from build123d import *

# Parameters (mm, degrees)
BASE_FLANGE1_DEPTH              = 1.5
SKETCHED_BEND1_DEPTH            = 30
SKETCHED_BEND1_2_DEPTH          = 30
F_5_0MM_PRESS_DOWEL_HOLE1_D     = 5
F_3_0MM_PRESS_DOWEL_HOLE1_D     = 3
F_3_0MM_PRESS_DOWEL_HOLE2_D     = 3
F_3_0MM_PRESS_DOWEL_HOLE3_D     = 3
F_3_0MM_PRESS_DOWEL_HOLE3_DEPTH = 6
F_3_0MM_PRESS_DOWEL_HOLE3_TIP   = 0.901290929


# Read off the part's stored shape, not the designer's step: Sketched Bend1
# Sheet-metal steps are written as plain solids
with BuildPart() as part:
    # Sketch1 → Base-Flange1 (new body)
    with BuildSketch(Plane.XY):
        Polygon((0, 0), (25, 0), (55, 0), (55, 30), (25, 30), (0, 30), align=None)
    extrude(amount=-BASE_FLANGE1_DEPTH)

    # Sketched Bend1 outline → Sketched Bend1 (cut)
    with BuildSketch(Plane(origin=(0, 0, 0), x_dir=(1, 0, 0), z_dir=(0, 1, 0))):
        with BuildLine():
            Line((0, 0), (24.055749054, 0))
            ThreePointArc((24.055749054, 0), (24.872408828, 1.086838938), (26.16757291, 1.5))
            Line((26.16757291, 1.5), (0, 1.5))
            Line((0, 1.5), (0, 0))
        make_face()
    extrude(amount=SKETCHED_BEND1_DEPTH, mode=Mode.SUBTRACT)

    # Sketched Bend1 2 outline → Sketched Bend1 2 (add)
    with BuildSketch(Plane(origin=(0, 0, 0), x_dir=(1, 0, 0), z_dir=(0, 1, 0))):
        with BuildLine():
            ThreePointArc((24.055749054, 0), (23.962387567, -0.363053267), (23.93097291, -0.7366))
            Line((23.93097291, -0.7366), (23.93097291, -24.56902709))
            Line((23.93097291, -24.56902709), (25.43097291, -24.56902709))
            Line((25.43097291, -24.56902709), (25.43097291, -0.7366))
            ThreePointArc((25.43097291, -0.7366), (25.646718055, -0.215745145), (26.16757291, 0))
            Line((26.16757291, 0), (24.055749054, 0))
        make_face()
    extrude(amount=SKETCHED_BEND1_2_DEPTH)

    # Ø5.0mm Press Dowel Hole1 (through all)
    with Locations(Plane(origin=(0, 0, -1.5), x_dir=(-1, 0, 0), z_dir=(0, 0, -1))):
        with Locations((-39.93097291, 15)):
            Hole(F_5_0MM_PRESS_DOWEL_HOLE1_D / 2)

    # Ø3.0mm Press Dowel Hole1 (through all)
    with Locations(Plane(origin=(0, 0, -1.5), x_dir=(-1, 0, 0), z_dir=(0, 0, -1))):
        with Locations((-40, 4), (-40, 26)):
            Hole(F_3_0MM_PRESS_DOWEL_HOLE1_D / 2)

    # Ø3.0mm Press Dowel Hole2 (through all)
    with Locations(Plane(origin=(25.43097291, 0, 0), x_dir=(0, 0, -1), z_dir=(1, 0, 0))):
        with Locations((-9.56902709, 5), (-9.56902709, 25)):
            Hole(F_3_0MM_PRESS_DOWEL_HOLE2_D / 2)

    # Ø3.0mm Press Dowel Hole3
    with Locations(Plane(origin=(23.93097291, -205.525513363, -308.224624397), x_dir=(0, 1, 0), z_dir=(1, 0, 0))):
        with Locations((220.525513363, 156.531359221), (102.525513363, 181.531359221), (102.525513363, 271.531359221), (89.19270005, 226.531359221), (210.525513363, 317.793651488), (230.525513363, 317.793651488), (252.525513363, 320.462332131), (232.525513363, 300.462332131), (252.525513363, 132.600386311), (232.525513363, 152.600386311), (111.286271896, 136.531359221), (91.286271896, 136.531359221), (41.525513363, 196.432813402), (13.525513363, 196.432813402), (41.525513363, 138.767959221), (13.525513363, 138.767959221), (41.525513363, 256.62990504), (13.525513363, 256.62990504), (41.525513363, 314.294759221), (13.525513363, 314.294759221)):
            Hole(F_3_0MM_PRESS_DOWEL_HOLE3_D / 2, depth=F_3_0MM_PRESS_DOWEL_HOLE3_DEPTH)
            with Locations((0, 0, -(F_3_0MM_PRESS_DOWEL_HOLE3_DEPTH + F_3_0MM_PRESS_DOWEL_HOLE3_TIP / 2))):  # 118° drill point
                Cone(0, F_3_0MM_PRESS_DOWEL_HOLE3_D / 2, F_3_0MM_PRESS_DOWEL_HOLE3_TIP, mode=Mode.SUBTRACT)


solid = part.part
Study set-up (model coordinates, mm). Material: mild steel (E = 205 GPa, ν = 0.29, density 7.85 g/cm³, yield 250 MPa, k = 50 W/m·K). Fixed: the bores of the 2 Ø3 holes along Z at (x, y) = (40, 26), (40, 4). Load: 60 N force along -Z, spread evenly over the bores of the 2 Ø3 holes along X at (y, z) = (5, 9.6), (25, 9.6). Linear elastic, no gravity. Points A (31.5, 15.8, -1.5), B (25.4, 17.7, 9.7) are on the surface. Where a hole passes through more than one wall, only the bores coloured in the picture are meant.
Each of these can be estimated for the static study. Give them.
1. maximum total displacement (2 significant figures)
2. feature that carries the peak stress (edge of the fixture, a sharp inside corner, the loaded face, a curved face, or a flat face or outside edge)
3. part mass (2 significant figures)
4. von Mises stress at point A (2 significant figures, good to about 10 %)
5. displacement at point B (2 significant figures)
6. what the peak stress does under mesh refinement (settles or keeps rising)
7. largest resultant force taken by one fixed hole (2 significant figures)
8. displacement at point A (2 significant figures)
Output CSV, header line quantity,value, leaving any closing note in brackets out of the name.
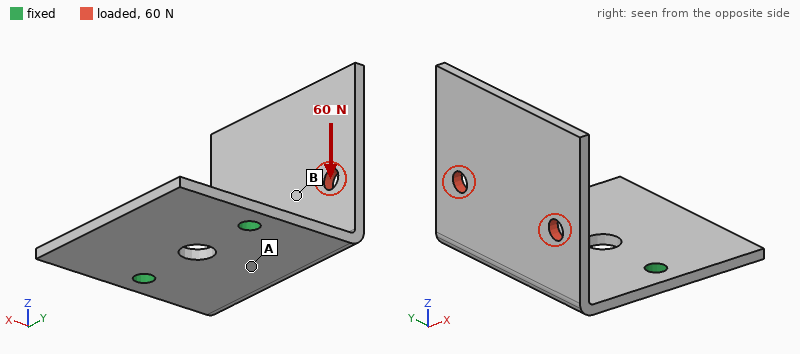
quantity,value
maximum total displacement,0.11 mm
feature that carries the peak stress,edge of the fixture
part mass,19 g
von Mises stress at point A,30 MPa
displacement at point B,0.057 mm
what the peak stress does under mesh refinement,keeps rising
largest resultant force taken by one fixed hole,30 N
displacement at point A,0.018 mm
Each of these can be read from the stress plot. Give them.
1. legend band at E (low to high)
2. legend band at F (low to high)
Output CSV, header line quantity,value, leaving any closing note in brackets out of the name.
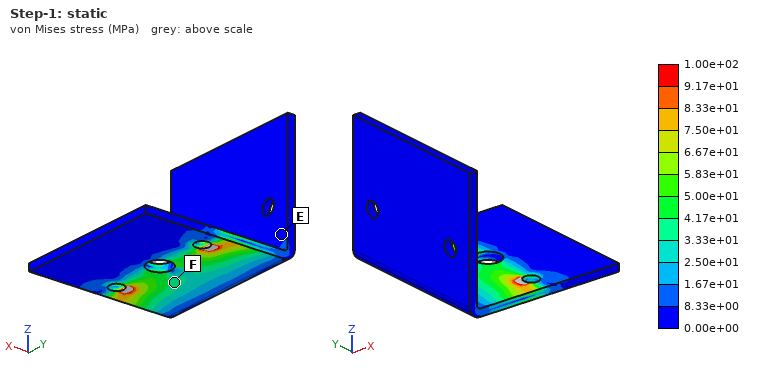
quantity,value
legend band at E,0.00e+00 to 8.33e+00 MPa
legend band at F,3.33e+01 to 4.17e+01 MPa
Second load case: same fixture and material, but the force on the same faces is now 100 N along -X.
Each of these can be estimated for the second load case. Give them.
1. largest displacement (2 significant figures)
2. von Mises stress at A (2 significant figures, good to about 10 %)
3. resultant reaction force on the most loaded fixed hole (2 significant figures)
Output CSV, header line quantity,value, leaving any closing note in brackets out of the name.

quantity,value
largest displacement,0.29 mm
von Mises stress at A,75 MPa
resultant reaction force on the most loaded fixed hole,51 N
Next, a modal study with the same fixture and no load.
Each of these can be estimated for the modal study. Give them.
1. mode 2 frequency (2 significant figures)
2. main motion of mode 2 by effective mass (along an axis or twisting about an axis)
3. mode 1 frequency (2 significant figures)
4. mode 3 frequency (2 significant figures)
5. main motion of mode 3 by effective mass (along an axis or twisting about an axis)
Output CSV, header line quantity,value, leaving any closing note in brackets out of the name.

quantity,value
mode 2 frequency,2000 Hz
main motion of mode 2 by effective mass,along Y
mode 1 frequency,980 Hz
mode 3 frequency,3000 Hz
main motion of mode 3 by effective mass,along Z
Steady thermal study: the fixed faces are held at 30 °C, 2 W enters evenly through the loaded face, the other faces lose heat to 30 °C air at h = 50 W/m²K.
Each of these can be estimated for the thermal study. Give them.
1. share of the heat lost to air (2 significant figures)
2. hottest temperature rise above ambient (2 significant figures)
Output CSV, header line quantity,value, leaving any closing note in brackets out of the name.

quantity,value
share of the heat lost to air,55 %
hottest temperature rise above ambient,15 K
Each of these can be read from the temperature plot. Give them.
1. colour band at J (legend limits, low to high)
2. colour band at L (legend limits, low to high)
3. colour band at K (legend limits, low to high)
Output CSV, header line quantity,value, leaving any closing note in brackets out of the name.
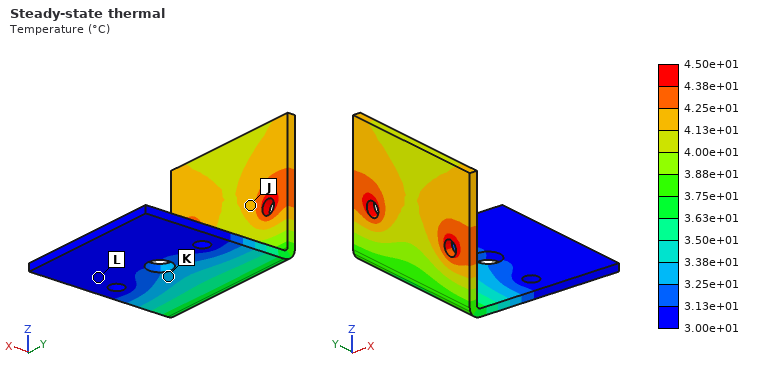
quantity,value
colour band at J,4.13e+01 to 4.25e+01 °C
colour band at L,3.00e+01 to 3.13e+01 °C
colour band at K,3.25e+01 to 3.38e+01 °C
